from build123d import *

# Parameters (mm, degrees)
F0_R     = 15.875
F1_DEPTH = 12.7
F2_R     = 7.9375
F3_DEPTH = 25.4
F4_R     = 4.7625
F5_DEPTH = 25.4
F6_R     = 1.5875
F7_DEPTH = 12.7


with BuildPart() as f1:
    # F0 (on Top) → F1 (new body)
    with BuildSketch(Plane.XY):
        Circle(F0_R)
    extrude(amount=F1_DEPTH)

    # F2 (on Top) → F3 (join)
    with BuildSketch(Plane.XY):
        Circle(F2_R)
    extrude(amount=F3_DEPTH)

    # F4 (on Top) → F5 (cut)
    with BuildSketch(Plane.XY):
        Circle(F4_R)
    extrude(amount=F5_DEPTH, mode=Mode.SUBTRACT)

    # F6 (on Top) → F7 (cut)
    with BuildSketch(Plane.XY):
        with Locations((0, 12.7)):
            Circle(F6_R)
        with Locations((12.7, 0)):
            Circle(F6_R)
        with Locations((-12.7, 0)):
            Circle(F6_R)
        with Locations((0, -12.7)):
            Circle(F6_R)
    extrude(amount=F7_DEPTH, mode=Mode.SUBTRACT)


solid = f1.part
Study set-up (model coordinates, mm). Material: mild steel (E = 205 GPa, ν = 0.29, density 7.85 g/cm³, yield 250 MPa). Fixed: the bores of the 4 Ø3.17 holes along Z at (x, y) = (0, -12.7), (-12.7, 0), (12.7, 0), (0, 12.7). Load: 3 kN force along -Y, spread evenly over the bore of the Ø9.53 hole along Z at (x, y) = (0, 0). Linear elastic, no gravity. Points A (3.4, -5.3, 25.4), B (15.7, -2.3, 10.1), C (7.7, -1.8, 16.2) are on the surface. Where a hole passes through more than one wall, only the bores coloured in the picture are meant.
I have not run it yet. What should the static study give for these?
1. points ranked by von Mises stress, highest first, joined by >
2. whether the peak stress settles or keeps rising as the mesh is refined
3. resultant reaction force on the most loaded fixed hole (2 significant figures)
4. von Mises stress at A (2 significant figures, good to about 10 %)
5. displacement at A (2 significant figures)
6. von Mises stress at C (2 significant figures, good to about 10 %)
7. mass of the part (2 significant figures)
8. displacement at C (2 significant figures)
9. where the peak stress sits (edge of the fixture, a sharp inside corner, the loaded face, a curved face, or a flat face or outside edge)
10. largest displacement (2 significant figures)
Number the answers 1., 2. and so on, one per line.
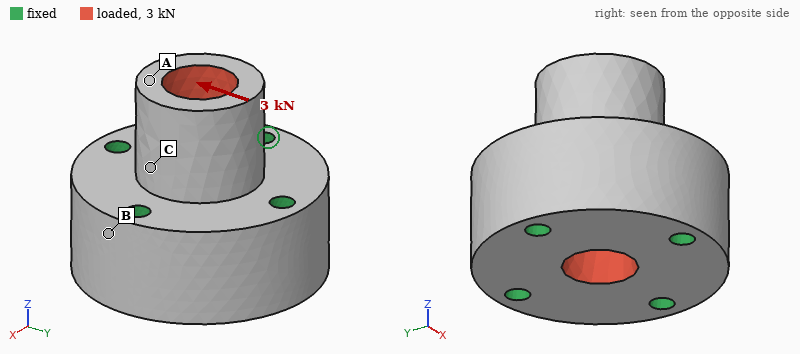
1. C > A > B
2. keeps rising
3. 1.1 kN
4. 9.8 MPa
5. 3.9 µm
6. 19 MPa
7. 81 g
8. 1.5 µm
9. a sharp inside corner
10. 4.0 µm
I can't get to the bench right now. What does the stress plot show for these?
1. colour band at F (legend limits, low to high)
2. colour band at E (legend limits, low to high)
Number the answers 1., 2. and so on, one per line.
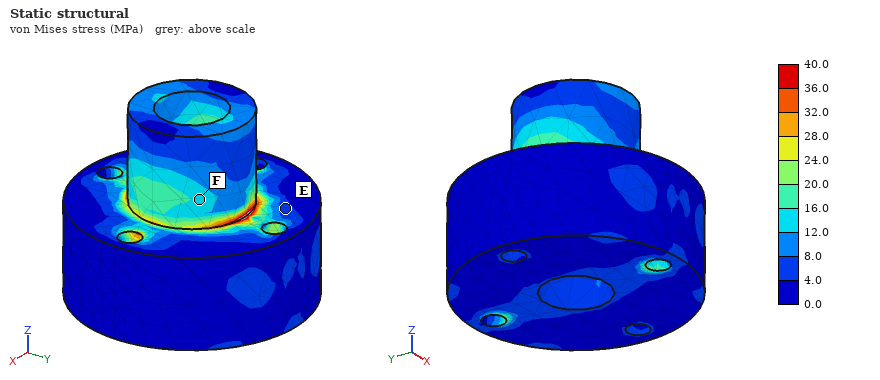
1. 12.0 to 16.0 MPa
2. 4.0 to 8.0 MPa
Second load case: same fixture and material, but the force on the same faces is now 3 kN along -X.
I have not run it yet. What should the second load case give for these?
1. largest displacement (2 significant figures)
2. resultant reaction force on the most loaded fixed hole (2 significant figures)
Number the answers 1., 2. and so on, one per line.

1. 4.1 µm
2. 1.1 kN
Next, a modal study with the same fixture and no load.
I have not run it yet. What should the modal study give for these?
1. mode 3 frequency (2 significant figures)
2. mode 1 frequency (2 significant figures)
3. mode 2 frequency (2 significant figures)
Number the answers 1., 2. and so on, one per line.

1. 53 kHz
2. 32 kHz
3. 32 kHz
